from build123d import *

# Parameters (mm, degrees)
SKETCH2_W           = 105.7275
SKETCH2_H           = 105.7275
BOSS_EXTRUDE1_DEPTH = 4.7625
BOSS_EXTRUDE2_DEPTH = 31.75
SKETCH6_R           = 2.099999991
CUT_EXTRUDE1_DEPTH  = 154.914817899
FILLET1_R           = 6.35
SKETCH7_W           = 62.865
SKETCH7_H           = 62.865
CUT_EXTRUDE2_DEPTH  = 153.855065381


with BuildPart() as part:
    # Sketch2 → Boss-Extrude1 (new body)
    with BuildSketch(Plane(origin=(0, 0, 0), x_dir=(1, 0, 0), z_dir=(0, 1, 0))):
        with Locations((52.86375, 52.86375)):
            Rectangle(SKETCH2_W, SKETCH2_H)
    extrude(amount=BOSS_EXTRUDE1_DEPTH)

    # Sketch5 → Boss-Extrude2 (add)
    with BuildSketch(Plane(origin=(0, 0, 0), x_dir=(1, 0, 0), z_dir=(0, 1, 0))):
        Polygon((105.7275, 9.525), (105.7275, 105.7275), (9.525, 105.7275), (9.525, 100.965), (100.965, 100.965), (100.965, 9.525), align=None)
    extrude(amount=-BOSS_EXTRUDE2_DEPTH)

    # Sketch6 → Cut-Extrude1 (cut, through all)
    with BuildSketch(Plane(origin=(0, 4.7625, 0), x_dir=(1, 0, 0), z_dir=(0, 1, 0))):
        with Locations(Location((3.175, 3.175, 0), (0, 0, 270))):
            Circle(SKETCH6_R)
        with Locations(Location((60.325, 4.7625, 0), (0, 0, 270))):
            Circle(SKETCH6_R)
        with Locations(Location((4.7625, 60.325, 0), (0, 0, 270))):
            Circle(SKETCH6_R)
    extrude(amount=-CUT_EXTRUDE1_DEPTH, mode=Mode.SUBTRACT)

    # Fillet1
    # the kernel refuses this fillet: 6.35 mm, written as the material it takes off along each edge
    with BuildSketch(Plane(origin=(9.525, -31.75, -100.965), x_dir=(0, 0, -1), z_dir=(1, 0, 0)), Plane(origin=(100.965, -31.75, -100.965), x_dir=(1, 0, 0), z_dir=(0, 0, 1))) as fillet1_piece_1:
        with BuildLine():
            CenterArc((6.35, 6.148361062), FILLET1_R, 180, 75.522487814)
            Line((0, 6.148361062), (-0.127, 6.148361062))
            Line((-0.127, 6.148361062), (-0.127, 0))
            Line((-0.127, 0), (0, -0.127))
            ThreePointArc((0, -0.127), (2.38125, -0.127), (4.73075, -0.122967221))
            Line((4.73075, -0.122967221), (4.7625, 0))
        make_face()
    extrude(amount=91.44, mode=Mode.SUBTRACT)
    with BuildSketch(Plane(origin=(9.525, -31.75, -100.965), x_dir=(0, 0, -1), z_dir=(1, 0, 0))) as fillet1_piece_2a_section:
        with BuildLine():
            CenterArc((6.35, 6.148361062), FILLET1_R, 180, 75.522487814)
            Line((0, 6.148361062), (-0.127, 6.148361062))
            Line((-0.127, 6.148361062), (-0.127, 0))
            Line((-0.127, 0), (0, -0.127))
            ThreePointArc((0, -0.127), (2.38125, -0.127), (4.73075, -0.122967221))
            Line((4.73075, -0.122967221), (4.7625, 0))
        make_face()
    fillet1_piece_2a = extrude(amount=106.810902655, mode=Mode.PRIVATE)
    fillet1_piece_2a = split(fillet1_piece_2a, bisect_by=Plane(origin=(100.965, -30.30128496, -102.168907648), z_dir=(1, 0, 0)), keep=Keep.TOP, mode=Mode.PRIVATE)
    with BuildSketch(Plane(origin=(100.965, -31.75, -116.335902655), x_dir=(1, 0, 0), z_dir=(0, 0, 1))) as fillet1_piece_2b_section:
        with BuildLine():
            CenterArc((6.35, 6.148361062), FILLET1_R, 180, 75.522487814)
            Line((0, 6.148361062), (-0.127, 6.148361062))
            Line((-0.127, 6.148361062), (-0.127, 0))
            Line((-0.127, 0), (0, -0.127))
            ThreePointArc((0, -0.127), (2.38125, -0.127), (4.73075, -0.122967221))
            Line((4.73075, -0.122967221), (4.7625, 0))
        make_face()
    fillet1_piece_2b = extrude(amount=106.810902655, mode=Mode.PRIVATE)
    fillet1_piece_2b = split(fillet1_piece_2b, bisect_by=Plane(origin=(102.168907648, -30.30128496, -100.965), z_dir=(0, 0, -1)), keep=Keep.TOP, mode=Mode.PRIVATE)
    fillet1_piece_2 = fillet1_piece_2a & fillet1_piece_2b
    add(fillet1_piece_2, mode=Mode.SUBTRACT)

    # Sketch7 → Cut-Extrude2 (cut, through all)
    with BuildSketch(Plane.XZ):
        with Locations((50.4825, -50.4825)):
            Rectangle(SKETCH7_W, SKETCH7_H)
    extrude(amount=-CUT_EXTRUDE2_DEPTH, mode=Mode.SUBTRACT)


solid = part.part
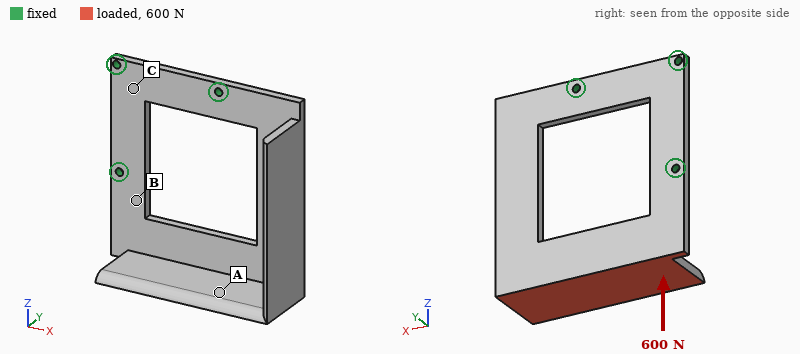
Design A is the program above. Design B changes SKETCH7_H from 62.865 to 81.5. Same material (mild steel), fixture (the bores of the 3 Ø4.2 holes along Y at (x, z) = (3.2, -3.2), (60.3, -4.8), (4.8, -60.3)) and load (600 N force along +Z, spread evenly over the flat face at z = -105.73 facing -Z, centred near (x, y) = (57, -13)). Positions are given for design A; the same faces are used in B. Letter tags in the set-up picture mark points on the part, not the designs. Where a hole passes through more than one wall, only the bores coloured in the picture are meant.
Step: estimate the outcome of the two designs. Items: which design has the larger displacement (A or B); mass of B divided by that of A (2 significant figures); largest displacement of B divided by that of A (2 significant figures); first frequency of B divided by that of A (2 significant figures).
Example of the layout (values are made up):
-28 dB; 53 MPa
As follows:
B; 0.91; 1.3; 0.85
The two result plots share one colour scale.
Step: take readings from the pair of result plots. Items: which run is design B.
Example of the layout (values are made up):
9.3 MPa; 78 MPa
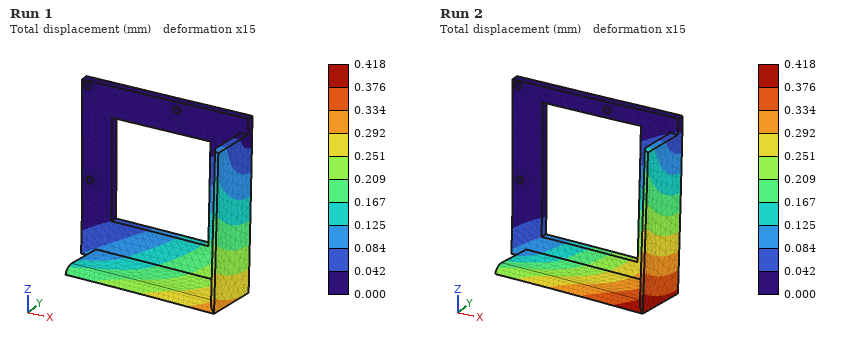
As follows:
Run 2
